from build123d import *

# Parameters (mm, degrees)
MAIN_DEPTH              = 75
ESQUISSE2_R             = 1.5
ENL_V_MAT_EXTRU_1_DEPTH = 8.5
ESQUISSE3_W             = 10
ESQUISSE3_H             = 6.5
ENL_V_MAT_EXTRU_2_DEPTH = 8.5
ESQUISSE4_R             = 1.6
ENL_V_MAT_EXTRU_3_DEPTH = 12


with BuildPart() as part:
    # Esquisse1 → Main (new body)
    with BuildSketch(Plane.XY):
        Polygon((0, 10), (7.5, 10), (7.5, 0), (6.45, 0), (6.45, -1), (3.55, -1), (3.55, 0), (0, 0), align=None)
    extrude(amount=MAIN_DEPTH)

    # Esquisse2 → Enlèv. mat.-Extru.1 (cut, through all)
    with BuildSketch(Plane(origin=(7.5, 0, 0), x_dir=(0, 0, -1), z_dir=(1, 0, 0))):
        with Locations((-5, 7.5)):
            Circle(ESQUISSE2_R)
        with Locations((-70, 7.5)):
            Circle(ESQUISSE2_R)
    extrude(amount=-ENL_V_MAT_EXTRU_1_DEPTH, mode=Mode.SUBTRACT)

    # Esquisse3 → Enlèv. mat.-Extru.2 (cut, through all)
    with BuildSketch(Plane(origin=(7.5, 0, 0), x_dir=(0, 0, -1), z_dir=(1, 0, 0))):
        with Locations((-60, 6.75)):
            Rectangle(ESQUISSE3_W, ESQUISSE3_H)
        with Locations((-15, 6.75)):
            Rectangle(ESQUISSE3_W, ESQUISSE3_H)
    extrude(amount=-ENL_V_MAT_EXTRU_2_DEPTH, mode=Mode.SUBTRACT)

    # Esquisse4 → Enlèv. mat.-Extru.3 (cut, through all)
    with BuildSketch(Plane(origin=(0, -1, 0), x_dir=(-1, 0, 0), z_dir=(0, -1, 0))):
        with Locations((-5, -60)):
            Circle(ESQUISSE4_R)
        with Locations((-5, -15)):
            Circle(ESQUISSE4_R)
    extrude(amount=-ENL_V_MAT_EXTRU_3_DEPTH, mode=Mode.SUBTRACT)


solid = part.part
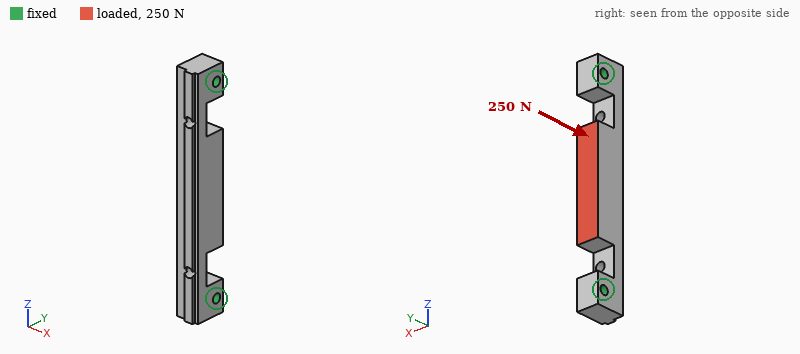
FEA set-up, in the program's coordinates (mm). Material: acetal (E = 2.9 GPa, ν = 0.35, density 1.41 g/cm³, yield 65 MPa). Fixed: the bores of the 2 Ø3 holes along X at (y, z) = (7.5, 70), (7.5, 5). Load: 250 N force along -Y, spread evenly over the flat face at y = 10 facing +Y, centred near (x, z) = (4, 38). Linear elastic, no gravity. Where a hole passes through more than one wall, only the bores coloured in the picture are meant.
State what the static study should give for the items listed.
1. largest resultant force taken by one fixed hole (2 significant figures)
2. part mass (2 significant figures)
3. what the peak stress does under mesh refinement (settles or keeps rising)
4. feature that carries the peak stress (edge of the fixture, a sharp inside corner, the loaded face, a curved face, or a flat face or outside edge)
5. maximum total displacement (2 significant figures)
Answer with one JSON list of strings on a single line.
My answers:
["130 N", "6.6 g", "keeps rising", "a sharp inside corner", "0.58 mm"]
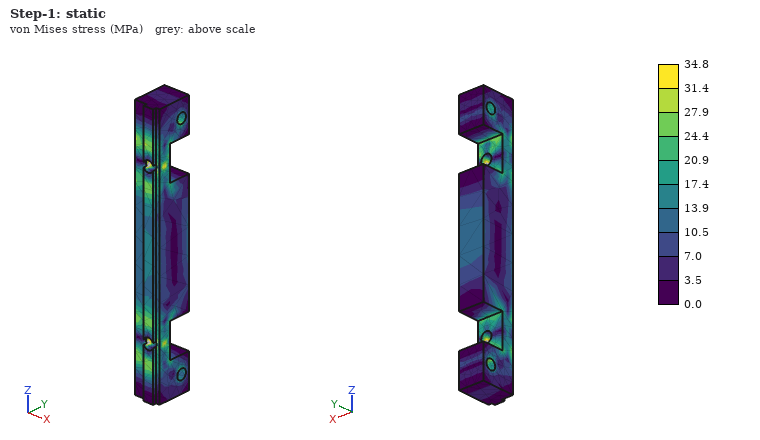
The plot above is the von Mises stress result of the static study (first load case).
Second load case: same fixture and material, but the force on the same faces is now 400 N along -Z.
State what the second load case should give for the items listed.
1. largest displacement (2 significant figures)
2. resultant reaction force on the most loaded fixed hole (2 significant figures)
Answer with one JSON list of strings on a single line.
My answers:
["0.31 mm", "210 N"]
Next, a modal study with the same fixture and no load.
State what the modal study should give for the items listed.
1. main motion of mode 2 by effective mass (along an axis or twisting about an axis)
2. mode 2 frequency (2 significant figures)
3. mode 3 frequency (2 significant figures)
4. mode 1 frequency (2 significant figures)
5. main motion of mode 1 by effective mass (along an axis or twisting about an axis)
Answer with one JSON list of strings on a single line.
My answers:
["along Y", "1700 Hz", "2900 Hz", "1400 Hz", "along X"]
